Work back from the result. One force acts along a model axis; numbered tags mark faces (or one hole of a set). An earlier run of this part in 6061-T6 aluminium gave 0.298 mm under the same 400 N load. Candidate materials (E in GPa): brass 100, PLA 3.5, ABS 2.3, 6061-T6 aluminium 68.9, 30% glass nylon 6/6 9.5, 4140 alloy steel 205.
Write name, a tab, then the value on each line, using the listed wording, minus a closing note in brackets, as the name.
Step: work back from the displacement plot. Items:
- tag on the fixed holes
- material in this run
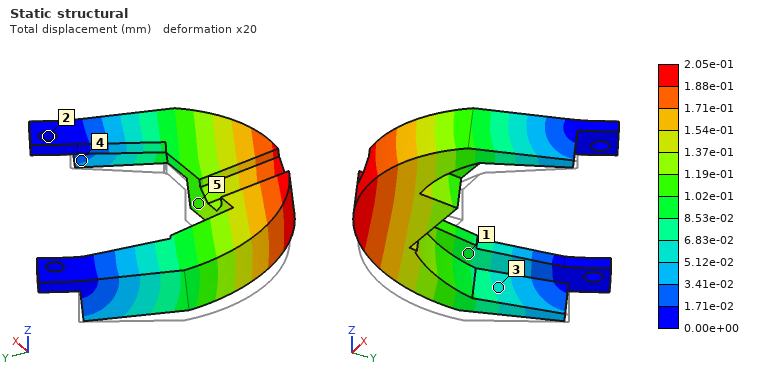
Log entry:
tag on the fixed holes	2
material in this run	brass
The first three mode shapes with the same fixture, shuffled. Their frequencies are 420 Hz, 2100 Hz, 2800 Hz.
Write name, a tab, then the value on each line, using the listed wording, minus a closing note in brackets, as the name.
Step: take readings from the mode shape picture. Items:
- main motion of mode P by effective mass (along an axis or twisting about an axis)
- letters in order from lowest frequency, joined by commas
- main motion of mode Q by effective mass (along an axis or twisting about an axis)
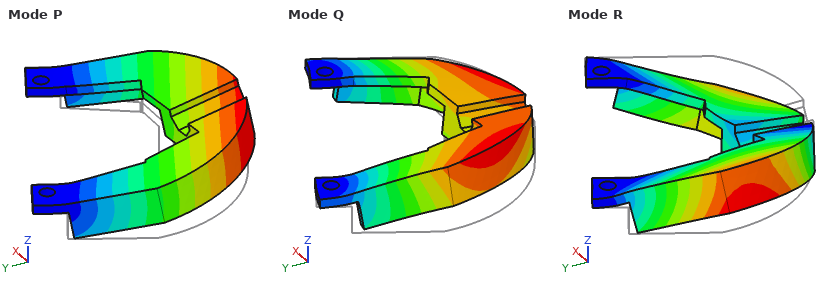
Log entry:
main motion of mode P by effective mass	along Z
letters in order from lowest frequency, joined by commas	P, R, Q
main motion of mode Q by effective mass	along X
